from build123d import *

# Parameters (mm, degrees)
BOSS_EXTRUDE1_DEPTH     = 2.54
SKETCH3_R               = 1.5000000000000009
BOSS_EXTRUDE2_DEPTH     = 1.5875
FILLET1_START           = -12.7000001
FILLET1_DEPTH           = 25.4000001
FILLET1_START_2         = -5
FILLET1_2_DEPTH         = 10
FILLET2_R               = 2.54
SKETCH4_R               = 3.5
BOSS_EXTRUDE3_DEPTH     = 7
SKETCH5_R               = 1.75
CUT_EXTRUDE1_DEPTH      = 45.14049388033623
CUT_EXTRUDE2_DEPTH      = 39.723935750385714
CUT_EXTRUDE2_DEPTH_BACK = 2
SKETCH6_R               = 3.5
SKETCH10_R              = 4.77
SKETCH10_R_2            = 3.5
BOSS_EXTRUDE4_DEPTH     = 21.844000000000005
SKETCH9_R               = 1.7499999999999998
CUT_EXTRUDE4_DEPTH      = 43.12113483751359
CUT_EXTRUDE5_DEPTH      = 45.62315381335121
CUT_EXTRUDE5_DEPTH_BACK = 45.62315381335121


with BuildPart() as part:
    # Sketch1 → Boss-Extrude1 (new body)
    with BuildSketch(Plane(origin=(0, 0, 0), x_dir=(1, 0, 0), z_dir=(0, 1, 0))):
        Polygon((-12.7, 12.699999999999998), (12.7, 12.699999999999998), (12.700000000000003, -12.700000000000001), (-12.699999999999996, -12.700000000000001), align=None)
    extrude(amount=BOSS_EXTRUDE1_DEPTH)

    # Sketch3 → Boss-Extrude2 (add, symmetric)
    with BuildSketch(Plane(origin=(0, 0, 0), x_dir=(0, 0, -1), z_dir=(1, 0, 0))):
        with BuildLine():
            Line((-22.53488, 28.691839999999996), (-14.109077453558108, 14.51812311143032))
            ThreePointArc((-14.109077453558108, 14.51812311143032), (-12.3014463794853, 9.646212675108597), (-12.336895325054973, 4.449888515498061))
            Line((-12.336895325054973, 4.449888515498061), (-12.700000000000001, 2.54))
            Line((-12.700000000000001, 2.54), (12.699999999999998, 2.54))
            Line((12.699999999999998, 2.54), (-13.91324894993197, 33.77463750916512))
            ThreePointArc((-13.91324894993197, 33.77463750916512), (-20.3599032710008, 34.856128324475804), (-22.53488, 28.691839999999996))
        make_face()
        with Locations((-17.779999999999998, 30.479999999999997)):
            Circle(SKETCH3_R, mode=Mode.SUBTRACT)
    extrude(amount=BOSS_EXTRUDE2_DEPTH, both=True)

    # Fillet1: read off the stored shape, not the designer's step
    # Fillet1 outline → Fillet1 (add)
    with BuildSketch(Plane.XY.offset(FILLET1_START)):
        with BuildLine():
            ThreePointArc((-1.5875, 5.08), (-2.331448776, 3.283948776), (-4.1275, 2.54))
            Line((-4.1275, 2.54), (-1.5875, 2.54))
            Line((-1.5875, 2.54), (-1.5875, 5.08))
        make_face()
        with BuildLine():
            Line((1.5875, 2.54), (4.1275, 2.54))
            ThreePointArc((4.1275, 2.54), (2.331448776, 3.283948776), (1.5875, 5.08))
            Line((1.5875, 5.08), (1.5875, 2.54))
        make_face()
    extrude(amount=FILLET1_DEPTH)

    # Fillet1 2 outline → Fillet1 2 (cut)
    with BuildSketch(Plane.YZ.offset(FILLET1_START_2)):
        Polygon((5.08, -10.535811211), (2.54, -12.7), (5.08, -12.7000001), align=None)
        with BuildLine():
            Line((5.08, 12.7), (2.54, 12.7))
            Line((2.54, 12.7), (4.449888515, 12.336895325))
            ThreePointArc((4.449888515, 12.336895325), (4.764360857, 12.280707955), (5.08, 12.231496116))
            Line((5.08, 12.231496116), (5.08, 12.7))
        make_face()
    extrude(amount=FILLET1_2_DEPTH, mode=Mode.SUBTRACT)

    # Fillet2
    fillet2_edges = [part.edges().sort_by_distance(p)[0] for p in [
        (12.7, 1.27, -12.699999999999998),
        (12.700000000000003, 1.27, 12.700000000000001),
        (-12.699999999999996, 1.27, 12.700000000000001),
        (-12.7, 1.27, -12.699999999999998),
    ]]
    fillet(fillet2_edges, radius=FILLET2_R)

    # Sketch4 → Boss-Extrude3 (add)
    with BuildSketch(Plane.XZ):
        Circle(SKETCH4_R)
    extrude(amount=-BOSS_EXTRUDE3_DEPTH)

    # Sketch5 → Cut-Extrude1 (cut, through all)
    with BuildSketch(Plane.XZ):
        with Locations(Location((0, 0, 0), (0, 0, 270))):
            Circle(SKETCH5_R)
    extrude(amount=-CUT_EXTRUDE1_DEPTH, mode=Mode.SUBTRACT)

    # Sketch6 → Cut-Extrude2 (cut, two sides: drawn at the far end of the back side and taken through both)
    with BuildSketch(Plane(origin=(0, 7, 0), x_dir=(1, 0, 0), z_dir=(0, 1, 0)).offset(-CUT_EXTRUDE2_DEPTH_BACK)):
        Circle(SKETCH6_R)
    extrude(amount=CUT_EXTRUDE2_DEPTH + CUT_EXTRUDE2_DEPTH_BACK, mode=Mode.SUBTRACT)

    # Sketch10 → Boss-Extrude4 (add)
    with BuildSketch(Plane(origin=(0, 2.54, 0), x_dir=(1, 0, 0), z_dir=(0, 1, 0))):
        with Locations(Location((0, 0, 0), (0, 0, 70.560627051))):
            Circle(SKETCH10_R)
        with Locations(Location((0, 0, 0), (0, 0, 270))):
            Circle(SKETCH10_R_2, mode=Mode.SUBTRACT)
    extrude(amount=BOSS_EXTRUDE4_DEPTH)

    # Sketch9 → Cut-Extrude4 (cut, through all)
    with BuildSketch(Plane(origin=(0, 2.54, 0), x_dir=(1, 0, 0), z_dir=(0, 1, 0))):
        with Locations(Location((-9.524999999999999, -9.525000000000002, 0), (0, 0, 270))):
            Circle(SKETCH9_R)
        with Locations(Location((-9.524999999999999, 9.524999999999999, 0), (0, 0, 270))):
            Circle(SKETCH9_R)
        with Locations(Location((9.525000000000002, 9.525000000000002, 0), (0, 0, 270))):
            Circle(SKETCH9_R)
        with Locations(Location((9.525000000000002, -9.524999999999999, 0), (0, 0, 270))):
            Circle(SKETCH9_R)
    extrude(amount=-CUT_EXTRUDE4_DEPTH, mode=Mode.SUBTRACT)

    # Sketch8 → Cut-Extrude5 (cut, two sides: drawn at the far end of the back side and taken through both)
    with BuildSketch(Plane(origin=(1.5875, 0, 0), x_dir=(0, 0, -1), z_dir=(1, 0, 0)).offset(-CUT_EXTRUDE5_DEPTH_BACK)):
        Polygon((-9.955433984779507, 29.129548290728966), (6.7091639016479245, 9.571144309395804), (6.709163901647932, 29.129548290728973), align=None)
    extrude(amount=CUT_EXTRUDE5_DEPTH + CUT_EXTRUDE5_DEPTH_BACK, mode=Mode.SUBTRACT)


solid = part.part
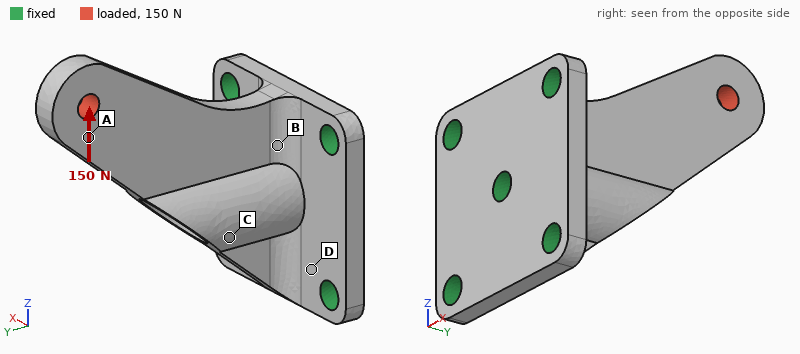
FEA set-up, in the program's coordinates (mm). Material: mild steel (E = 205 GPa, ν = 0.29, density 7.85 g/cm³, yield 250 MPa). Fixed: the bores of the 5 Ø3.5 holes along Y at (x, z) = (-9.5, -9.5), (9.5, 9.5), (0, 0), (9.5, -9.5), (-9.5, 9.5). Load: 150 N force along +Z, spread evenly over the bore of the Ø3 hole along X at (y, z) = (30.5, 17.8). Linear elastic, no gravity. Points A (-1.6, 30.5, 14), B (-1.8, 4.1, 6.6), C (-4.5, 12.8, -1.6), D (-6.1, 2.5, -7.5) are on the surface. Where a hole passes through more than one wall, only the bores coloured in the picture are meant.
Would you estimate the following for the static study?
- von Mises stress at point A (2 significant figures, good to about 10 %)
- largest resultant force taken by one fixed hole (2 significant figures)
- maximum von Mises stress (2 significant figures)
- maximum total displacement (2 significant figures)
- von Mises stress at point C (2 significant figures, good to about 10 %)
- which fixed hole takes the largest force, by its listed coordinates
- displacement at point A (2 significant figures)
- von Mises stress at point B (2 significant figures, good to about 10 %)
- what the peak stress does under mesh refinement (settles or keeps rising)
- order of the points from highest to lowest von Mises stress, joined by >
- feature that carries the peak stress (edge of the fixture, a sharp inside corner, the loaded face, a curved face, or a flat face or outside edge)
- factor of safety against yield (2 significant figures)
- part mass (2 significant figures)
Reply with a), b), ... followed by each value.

a) 8.9 MPa
b) 240 N
c) 83 MPa
d) 18 µm
e) 31 MPa
f) (0, 0)
g) 14 µm
h) 17 MPa
i) settles
j) C > B > A > D
k) a curved face
l) 3.0
m) 26 g
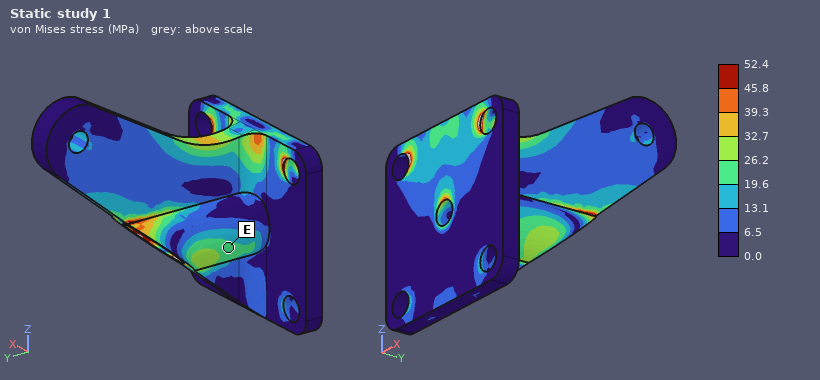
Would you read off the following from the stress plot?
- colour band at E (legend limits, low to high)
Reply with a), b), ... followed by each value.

a) 19.6 to 26.2 MPa
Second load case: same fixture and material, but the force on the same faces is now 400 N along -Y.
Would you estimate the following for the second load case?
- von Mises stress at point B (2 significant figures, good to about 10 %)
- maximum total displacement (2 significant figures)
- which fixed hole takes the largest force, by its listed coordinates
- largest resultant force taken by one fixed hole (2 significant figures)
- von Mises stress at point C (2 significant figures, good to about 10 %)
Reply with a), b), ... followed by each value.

a) 35 MPa
b) 29 µm
c) (0, 0)
d) 230 N
e) 39 MPa
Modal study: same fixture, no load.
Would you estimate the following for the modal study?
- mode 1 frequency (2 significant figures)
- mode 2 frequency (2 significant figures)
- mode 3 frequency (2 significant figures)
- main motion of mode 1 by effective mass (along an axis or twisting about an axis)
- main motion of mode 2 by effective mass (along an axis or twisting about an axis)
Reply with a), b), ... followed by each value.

a) 3900 Hz
b) 7900 Hz
c) 14 kHz
d) along X
e) along Z
